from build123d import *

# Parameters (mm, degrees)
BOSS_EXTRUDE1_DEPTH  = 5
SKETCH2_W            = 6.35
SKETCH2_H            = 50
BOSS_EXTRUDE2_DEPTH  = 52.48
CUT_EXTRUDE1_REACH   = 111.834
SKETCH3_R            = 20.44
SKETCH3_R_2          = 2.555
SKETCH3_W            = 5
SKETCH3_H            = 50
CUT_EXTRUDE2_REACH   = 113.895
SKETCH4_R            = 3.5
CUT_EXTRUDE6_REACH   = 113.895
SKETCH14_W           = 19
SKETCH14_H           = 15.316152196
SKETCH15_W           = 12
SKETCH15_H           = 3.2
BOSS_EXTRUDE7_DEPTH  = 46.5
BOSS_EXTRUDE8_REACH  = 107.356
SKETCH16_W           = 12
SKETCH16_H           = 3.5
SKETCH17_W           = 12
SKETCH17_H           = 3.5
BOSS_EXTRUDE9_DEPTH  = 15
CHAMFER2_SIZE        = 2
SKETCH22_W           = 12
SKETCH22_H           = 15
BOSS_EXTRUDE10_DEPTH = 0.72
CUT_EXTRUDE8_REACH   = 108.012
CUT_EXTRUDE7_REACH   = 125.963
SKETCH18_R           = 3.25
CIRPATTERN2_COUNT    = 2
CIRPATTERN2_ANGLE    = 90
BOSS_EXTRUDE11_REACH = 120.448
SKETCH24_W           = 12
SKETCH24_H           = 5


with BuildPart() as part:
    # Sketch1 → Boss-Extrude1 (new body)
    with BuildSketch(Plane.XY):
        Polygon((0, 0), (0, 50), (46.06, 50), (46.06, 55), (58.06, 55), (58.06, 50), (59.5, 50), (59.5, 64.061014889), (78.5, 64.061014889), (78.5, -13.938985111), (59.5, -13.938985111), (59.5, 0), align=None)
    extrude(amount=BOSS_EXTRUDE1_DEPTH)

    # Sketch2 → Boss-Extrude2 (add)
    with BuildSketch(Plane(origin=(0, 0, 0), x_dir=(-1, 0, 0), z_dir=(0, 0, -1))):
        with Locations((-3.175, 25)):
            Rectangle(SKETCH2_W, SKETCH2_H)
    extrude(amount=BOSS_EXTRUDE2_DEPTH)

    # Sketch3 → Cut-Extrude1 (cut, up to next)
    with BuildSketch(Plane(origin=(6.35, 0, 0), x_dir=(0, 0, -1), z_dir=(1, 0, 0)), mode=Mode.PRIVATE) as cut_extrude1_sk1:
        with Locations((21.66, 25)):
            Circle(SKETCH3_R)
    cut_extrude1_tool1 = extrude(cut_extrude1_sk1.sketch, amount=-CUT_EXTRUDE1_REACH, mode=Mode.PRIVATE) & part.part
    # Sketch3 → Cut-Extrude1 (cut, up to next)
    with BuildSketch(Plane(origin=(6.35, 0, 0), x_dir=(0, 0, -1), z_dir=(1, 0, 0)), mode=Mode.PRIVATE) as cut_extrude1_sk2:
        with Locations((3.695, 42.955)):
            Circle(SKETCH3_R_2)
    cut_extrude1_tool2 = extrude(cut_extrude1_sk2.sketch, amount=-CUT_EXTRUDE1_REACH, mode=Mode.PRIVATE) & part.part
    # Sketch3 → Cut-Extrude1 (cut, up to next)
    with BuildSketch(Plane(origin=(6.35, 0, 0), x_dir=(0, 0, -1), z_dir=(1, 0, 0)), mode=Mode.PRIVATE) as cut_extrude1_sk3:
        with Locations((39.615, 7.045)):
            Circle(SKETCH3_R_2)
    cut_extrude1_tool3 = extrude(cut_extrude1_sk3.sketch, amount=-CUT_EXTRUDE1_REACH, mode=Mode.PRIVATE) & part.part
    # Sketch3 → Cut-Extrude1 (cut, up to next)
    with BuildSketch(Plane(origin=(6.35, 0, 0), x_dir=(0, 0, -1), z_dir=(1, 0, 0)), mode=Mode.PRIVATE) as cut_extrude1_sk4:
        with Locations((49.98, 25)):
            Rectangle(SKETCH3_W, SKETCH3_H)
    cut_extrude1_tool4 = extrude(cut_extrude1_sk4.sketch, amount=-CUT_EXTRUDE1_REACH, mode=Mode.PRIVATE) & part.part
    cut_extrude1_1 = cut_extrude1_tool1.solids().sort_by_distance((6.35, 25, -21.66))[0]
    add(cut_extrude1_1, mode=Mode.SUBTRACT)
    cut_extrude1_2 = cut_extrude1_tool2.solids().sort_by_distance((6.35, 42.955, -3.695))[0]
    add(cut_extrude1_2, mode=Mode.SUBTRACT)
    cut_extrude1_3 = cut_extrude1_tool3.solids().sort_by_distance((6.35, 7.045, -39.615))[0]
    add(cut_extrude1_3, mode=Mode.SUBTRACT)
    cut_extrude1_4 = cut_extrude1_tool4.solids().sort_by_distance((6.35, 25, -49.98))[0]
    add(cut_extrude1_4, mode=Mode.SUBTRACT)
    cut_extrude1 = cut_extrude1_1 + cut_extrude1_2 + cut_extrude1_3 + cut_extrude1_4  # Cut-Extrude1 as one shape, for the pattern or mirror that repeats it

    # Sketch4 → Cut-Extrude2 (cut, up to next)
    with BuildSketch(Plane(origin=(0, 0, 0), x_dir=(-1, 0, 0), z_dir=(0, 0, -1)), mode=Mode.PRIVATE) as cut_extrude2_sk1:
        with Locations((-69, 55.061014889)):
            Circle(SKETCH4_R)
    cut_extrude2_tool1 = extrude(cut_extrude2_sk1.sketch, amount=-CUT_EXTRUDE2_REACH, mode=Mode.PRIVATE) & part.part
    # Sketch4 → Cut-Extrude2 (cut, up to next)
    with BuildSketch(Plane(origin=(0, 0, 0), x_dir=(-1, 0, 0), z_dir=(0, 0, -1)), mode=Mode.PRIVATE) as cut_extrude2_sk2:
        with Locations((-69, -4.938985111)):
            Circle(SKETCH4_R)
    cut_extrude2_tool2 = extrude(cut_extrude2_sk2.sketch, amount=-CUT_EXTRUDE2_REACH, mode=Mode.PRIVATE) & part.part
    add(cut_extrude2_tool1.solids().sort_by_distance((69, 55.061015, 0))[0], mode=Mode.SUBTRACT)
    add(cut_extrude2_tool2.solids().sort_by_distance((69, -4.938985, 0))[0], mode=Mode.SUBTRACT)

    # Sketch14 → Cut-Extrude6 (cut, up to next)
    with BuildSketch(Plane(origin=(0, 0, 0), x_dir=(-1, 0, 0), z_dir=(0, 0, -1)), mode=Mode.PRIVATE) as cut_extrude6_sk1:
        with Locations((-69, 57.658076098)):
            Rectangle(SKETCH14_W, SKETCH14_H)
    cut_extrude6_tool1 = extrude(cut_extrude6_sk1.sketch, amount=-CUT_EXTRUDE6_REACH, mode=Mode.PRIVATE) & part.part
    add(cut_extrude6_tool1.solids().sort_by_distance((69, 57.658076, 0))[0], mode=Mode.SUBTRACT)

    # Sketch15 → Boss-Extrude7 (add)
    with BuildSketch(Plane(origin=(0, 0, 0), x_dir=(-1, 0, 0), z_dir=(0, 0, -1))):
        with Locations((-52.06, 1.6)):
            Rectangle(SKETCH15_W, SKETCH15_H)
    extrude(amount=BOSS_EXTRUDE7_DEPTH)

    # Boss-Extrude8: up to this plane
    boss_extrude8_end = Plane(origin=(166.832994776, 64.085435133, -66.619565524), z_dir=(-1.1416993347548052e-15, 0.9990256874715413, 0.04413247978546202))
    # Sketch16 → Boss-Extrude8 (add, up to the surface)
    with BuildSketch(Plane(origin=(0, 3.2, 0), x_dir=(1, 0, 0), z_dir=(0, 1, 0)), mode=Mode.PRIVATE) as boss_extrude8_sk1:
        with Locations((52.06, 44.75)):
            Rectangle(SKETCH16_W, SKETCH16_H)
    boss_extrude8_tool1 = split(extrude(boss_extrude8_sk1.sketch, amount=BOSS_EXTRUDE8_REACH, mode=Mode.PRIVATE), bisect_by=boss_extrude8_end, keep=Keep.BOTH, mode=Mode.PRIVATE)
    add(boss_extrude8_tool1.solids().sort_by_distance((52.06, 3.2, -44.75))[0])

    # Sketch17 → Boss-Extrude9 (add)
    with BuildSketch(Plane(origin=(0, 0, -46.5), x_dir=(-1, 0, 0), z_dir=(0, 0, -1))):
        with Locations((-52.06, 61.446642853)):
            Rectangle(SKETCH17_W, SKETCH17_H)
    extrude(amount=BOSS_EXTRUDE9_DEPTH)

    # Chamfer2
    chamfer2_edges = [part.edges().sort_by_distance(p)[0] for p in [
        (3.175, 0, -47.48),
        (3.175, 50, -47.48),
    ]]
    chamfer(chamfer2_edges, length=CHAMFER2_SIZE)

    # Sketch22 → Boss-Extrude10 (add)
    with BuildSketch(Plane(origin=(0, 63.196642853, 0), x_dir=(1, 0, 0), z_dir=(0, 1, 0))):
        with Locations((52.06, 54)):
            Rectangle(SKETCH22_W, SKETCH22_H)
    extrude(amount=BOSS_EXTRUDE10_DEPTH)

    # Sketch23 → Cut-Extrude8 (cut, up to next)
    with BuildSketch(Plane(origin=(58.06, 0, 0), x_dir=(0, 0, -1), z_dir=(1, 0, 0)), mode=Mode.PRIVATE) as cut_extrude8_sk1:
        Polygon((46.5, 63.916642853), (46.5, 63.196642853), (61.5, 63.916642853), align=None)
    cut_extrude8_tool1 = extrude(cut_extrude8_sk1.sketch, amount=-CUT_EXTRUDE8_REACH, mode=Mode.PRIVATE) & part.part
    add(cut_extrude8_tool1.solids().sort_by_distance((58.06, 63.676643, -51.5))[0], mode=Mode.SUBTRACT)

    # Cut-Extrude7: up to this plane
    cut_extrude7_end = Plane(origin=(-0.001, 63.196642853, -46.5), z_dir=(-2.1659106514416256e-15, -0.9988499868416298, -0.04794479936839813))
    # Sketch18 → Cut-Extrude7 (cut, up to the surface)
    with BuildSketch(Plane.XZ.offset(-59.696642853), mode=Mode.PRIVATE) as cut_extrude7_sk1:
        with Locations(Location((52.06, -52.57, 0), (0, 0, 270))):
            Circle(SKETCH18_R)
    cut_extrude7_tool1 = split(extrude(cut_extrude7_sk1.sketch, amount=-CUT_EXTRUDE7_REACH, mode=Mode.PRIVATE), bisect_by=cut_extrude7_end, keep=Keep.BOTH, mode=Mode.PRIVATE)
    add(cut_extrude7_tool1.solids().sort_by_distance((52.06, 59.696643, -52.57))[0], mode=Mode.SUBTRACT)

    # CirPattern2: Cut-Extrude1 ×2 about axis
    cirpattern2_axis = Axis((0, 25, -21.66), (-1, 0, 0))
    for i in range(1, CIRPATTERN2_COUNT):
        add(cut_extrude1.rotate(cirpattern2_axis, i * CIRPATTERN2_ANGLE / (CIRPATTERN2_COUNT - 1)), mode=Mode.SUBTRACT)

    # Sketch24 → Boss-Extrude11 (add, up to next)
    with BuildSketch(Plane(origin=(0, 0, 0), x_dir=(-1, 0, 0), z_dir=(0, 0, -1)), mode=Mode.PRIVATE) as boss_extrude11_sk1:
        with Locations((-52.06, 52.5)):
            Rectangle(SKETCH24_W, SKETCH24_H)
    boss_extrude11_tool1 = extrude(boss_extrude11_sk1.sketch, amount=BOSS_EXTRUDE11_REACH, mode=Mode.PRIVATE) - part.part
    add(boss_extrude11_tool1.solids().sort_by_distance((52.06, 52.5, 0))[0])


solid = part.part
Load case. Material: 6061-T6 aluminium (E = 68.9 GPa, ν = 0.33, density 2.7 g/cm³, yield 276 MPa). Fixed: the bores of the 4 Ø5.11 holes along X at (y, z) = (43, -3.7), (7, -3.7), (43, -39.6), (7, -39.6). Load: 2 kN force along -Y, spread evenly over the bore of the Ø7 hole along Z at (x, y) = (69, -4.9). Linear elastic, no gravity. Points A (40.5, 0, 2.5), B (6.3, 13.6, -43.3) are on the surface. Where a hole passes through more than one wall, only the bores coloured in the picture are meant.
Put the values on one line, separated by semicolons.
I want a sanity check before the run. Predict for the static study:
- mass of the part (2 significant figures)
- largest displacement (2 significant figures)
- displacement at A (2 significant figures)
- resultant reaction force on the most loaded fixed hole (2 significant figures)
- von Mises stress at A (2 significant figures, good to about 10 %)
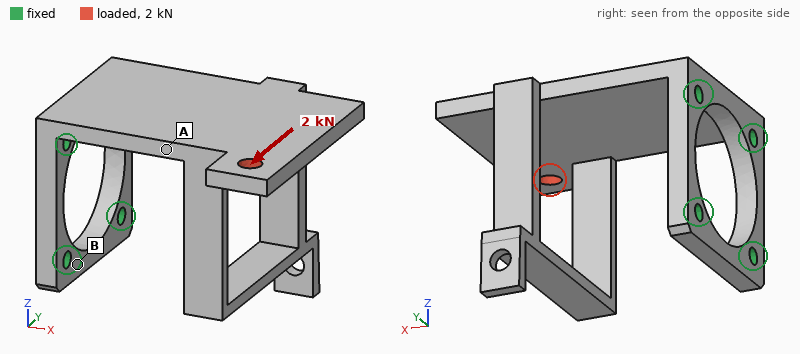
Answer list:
94 g; 0.22 mm; 0.084 mm; 3.6 kN; 30 MPa
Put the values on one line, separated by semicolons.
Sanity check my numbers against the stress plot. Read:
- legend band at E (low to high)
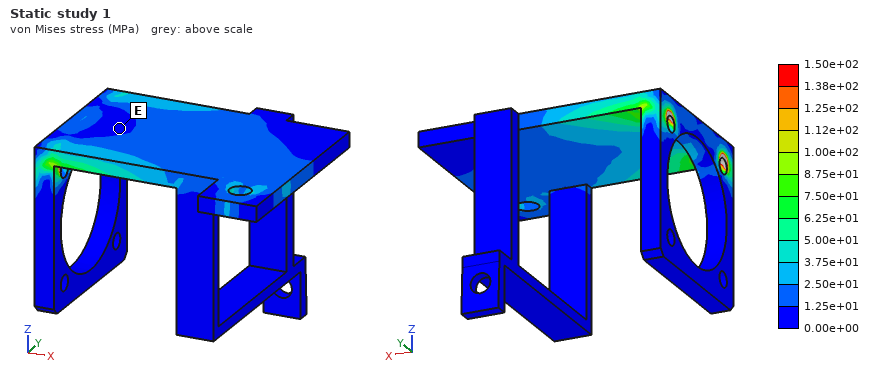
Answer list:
0.00e+00 to 1.25e+01 MPa
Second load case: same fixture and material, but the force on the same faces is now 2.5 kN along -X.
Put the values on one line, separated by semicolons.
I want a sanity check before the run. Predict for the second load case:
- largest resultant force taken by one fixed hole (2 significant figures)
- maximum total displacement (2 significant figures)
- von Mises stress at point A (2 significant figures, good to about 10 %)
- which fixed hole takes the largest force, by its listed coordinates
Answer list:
3.2 kN; 0.20 mm; 50 MPa; (7, -3.7)
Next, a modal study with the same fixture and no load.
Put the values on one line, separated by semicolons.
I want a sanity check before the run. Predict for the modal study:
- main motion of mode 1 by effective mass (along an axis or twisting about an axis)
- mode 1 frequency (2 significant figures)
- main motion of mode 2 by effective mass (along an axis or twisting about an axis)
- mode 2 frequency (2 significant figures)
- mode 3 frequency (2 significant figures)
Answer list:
along Z; 440 Hz; along Y; 710 Hz; 1300 Hz
